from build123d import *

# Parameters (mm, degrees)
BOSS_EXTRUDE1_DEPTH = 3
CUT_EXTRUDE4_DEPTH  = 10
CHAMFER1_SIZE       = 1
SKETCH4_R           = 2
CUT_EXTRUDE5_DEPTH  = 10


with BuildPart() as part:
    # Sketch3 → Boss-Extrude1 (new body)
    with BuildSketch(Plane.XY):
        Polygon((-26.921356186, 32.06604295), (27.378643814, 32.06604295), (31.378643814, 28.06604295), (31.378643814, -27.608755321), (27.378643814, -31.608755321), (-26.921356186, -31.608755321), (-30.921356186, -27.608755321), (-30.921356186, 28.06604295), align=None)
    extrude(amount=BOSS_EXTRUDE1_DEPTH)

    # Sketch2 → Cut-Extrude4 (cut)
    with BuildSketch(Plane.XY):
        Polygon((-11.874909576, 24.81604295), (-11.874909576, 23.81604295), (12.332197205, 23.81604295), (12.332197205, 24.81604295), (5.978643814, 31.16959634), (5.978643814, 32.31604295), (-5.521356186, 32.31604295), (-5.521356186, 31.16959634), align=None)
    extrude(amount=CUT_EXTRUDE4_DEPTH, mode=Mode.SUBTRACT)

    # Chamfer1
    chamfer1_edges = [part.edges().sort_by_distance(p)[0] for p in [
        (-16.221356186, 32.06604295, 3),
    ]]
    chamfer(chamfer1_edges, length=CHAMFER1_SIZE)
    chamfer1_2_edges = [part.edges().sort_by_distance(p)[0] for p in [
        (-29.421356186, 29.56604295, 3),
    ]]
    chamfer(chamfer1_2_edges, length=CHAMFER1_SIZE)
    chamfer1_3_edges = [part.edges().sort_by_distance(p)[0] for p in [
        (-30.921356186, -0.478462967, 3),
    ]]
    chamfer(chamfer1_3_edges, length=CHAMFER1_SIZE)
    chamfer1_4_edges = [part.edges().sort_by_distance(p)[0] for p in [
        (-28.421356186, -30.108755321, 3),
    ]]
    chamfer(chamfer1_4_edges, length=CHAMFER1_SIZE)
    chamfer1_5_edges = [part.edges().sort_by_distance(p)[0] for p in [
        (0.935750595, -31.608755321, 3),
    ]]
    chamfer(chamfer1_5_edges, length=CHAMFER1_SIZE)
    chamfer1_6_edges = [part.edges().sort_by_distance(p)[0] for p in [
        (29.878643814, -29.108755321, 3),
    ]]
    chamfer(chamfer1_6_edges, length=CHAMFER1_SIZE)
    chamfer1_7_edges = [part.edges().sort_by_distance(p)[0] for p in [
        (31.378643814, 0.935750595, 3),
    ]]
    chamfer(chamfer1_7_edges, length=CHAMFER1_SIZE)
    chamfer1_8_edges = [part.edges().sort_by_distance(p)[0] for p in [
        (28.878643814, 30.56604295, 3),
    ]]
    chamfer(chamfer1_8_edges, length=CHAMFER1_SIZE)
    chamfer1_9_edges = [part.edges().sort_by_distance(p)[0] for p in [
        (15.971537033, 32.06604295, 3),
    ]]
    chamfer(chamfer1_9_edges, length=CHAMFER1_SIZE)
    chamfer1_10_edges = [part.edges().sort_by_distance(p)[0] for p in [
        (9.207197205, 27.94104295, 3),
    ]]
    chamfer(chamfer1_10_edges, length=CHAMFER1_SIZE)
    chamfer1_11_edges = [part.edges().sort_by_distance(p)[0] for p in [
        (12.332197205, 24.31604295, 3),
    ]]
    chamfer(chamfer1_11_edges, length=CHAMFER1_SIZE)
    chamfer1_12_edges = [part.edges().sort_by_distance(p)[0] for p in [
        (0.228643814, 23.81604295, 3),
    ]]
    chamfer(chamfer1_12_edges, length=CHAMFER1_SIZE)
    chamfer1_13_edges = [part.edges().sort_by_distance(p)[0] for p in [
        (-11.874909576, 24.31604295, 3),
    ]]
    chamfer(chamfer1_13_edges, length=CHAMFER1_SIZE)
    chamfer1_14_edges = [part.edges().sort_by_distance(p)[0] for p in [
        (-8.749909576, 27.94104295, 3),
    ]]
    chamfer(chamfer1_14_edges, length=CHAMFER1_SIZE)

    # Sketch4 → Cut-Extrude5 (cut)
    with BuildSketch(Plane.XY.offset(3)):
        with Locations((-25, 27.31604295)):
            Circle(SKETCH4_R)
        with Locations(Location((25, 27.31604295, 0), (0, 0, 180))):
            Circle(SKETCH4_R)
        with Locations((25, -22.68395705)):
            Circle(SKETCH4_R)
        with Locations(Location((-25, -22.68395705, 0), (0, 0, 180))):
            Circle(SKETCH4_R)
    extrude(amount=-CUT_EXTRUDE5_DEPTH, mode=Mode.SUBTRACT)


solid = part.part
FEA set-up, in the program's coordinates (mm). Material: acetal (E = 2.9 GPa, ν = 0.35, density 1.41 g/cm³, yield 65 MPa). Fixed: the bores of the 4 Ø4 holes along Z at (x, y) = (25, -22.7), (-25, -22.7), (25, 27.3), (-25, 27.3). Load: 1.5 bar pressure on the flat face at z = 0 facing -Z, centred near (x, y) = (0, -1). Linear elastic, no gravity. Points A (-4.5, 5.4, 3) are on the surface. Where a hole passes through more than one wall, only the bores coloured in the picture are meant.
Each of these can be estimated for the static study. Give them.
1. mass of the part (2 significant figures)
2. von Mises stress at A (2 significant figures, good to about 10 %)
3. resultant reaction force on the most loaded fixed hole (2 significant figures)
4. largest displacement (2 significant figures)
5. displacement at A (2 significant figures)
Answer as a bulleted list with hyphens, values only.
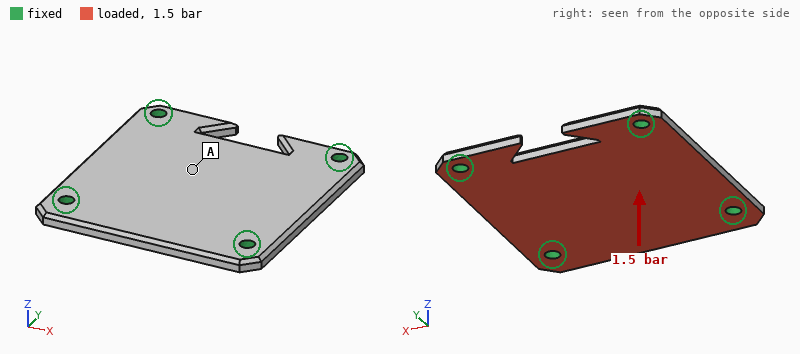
- 16 g
- 12 MPa
- 160 N
- 0.87 mm
- 0.85 mm
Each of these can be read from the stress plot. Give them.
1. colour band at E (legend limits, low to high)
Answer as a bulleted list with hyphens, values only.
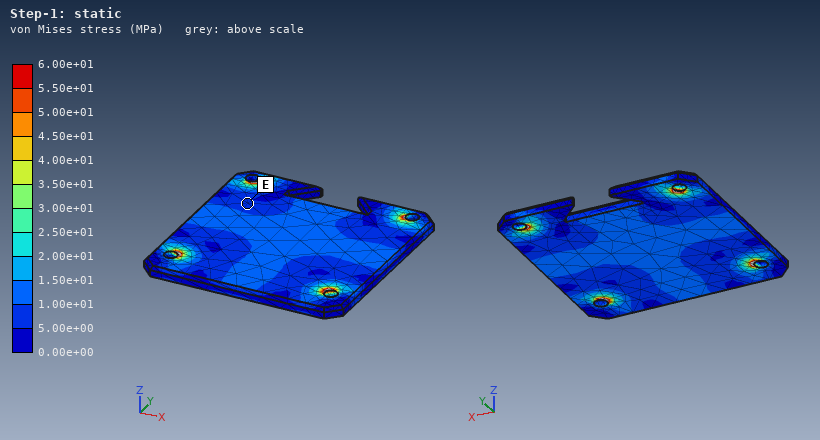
- 5.00e+00 to 1.00e+01 MPa
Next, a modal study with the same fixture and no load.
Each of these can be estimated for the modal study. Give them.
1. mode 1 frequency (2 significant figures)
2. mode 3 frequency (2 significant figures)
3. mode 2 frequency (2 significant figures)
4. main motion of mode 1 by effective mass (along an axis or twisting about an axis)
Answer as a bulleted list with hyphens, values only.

- 1200 Hz
- 2000 Hz
- 2000 Hz
- along Z
